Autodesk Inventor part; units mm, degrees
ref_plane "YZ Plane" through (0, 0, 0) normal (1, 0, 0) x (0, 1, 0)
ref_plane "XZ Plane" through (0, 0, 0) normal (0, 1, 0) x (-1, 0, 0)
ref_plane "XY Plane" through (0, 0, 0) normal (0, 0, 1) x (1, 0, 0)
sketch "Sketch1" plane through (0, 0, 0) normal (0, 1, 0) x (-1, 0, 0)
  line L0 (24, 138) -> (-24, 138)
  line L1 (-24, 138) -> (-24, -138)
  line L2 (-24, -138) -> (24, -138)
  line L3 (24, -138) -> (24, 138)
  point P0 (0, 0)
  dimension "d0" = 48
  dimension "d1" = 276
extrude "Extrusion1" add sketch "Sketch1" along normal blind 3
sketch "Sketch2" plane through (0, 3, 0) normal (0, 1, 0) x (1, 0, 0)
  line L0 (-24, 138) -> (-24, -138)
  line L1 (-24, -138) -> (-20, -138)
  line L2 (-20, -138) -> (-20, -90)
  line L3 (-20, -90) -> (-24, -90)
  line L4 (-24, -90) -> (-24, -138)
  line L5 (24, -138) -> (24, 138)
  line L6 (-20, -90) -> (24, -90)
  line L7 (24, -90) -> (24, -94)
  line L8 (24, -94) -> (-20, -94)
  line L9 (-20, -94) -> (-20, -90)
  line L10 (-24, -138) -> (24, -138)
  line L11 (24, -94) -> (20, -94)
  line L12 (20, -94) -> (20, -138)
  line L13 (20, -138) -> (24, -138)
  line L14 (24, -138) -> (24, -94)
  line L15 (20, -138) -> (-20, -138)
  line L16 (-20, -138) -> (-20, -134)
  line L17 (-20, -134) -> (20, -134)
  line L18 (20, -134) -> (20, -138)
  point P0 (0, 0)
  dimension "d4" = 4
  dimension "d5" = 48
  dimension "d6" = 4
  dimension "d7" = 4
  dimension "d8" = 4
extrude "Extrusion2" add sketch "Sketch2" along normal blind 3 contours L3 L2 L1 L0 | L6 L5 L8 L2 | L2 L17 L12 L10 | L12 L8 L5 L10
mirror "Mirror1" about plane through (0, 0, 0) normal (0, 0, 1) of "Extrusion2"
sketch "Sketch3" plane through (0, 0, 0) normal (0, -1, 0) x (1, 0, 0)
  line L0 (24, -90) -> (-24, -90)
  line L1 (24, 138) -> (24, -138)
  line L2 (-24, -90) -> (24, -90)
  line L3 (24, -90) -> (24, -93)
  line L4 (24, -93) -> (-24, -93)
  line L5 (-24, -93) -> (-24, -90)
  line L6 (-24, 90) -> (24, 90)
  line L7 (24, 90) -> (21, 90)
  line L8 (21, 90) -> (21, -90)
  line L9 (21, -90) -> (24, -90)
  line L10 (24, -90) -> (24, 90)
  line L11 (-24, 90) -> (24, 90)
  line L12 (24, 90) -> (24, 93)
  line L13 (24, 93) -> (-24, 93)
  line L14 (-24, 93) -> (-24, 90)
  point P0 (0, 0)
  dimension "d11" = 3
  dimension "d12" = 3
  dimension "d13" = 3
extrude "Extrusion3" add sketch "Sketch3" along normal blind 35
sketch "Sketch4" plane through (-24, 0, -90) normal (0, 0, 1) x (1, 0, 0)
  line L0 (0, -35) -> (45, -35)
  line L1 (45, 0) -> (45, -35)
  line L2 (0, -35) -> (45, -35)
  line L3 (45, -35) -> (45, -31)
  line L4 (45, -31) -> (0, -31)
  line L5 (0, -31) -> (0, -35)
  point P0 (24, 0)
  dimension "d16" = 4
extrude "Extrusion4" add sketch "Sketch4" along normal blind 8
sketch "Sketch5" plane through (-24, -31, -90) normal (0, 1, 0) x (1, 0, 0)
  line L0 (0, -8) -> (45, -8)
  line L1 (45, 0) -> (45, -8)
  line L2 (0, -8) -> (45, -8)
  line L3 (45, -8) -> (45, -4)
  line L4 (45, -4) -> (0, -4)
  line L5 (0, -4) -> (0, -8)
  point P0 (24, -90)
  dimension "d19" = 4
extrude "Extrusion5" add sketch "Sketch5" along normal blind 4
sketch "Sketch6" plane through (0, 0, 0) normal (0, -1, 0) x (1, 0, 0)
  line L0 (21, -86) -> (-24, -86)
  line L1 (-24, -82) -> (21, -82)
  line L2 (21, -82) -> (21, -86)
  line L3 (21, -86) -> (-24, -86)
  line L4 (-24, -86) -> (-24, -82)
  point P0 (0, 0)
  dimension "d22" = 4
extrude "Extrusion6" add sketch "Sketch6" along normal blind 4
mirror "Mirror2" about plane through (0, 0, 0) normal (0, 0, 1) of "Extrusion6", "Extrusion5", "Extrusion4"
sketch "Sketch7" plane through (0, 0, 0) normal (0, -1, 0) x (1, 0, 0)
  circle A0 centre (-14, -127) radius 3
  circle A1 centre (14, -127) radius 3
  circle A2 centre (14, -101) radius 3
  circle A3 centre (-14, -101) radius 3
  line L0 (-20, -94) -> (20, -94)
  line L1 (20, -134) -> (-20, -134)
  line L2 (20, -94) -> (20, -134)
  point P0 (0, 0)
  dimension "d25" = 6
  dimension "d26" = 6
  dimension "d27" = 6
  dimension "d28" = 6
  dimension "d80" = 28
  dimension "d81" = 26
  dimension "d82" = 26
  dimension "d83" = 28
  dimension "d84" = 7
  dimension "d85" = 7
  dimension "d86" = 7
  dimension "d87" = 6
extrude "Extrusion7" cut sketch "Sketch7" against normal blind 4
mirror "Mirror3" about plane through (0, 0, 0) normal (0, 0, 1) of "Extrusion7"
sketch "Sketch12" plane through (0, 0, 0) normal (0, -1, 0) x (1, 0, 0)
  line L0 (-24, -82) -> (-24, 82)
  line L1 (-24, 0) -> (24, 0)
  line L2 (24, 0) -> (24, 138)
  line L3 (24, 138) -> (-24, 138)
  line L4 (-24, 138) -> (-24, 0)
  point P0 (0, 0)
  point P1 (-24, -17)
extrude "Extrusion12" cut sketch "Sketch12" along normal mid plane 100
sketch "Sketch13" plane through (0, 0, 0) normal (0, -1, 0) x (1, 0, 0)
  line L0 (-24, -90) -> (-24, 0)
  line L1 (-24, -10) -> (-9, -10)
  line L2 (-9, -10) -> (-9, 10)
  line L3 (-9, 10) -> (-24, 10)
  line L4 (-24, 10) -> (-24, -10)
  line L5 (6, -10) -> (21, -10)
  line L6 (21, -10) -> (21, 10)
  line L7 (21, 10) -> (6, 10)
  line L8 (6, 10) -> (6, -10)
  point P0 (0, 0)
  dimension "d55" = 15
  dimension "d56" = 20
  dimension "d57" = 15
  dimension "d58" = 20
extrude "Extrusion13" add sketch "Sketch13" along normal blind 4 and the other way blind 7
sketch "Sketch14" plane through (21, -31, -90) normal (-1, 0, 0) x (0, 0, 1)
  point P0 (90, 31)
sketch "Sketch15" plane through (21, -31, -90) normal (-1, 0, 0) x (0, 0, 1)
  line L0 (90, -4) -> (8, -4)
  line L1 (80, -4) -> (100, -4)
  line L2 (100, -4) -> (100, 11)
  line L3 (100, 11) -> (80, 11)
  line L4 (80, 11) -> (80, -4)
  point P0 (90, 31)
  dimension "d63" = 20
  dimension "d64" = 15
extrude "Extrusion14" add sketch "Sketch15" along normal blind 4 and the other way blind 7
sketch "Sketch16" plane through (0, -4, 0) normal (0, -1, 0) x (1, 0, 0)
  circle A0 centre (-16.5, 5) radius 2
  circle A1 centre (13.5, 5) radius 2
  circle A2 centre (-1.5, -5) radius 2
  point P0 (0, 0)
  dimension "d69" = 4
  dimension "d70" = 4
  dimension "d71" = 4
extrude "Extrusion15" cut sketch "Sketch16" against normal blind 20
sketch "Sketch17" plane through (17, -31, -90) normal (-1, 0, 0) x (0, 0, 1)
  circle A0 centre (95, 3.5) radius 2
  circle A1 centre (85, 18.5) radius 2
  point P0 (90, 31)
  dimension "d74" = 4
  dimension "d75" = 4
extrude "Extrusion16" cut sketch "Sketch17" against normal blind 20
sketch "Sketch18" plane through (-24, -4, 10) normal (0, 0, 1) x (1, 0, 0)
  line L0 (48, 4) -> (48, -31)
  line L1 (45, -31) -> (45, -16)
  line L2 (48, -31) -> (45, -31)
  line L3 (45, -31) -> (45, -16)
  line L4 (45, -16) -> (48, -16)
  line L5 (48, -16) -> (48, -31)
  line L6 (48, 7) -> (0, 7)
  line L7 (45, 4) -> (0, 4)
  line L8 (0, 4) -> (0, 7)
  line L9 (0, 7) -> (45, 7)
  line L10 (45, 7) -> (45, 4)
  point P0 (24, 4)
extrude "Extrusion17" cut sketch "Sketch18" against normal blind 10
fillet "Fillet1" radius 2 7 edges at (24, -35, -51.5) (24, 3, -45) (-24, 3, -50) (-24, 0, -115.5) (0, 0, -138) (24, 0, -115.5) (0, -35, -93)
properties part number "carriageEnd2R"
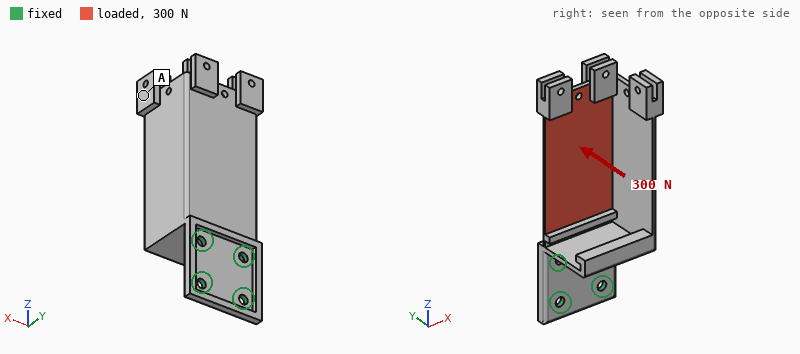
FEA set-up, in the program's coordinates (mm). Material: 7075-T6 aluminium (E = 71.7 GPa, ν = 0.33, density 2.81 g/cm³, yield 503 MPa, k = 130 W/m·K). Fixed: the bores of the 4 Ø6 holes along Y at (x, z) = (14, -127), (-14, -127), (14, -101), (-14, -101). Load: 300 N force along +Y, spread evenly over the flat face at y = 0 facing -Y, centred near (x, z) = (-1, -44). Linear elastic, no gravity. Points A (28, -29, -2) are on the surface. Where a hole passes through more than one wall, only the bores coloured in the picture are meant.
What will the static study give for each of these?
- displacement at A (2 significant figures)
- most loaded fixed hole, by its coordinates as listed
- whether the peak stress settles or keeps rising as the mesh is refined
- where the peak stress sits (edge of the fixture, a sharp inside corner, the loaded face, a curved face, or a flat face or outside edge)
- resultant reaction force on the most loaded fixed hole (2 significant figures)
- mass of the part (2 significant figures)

1.3 mm
(14, -101)
keeps rising
edge of the fixture
550 N
130 g
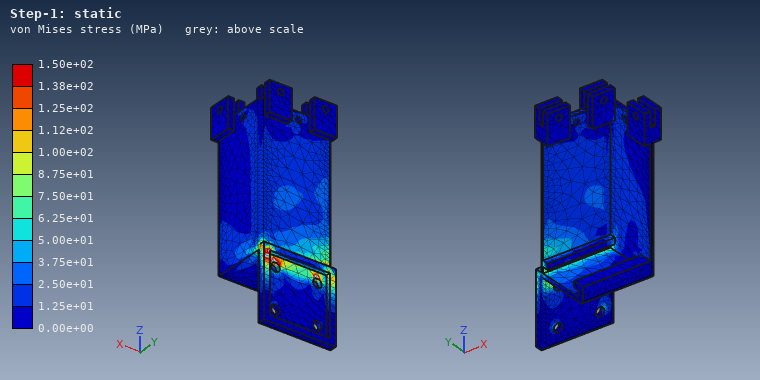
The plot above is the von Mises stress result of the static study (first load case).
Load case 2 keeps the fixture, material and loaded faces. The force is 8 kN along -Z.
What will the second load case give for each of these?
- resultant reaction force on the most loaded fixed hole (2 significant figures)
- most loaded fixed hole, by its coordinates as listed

3.9 kN
(-14, -101)
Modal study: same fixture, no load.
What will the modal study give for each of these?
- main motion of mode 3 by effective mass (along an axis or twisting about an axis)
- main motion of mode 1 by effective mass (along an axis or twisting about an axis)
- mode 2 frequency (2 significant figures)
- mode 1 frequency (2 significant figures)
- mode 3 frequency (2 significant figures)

along X
along Y
620 Hz
250 Hz
1400 Hz
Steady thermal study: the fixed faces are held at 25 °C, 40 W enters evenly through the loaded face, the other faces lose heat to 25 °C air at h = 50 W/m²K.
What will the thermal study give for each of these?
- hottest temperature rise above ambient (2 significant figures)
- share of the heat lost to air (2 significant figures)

40 K
57 %
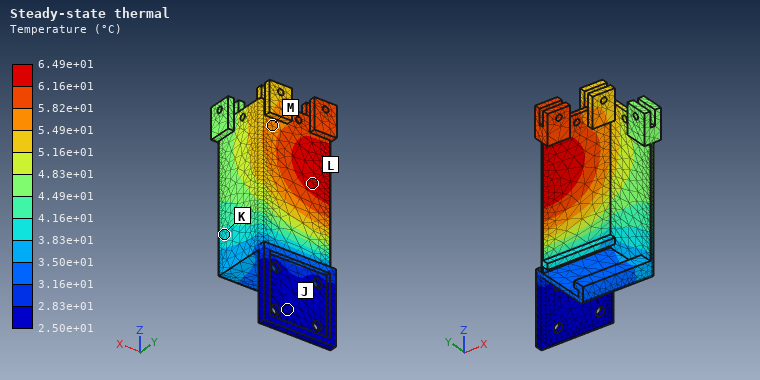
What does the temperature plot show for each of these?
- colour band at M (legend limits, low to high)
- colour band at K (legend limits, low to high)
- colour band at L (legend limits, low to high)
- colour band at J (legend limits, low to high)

5.49e+01 to 5.82e+01 °C
3.83e+01 to 4.16e+01 °C
6.16e+01 to 6.49e+01 °C
2.50e+01 to 2.83e+01 °C
